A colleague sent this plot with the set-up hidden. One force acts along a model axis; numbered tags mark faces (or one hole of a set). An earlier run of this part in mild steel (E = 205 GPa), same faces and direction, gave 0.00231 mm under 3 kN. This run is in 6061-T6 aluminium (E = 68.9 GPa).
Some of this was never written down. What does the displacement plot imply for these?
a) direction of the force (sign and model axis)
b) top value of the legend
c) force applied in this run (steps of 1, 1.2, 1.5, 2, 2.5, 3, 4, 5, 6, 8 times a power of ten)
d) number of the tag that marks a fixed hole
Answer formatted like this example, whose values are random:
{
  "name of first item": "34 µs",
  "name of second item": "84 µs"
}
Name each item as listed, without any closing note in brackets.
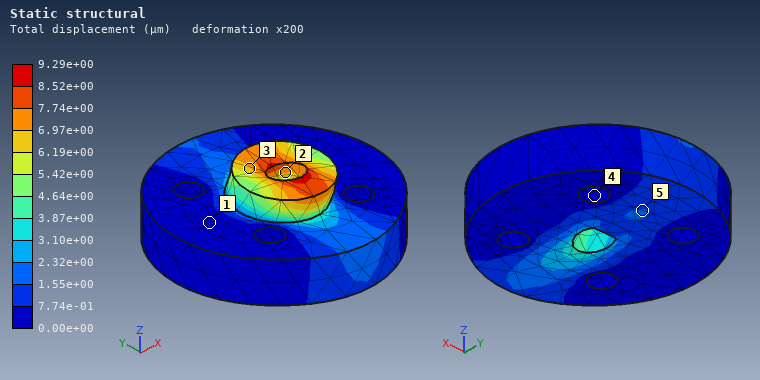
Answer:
{
  "direction of the force": "-Y",
  "top value of the legend": "9.29e+00 µm",
  "force applied in this run": "4 kN",
  "number of the tag that marks a fixed hole": "4"
}
